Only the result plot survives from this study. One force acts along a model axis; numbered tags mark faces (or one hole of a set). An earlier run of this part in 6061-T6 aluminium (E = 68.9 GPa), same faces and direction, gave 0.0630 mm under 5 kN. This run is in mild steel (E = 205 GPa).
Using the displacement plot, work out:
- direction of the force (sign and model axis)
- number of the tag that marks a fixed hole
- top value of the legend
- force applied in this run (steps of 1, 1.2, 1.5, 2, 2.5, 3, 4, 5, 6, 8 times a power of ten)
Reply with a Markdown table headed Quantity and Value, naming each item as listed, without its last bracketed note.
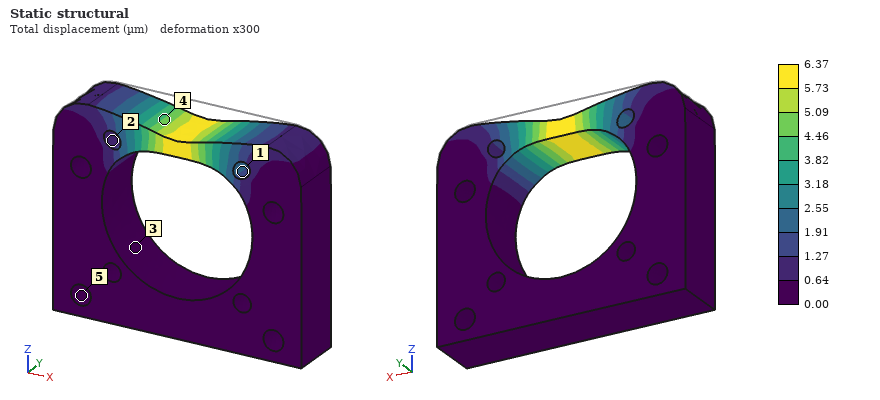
| Quantity | Value |
|---|---|
| direction of the force | -Z |
| number of the tag that marks a fixed hole | 5 |
| top value of the legend | 6.37 µm |
| force applied in this run | 1.5 kN |
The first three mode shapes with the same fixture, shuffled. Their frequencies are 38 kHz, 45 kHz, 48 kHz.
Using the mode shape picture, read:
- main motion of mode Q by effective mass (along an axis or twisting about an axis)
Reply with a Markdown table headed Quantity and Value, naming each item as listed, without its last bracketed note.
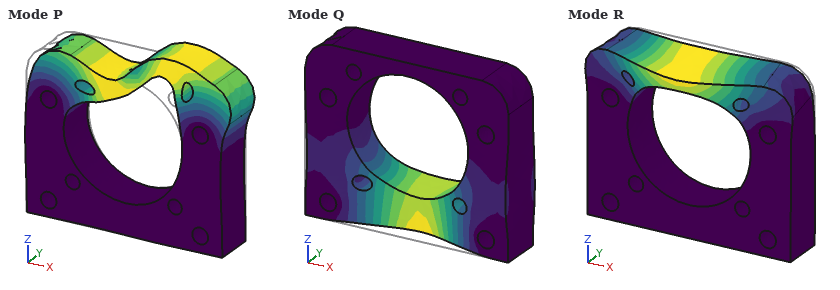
| Quantity | Value |
|---|---|
| main motion of mode Q by effective mass | along Y |
